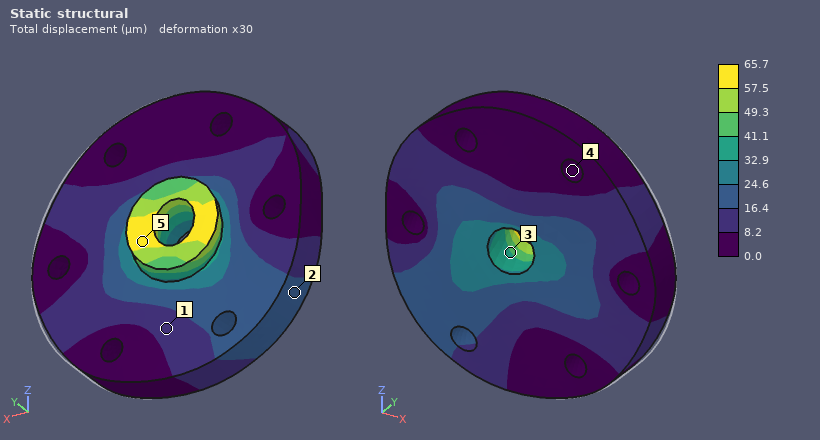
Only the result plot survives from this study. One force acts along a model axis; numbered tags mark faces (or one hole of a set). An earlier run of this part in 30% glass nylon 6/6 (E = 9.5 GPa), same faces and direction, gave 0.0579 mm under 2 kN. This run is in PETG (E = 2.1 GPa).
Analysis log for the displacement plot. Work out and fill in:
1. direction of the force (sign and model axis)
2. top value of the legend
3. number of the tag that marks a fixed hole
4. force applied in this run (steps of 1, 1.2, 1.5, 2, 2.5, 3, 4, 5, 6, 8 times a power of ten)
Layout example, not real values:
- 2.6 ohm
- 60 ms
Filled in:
- -X
- 65.7 µm
- 4
- 500 N
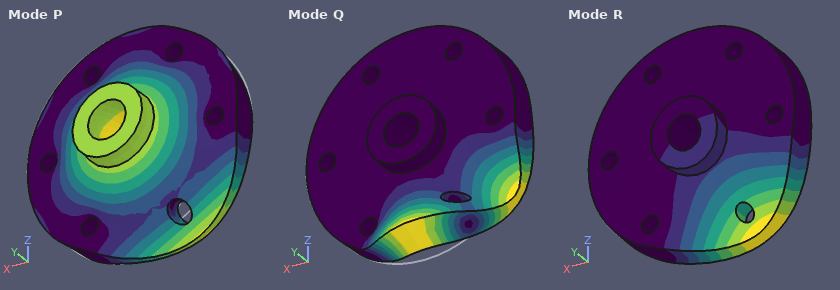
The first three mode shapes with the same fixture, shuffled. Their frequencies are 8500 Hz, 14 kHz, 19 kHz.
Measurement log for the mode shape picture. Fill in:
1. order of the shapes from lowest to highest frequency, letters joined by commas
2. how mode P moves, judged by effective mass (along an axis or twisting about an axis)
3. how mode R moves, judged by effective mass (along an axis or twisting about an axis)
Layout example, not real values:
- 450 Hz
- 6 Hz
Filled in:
- R, P, Q
- along Y
- along Y
